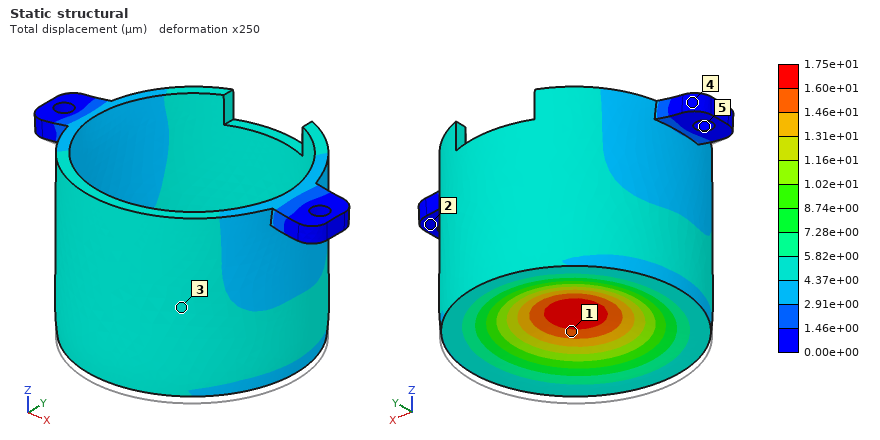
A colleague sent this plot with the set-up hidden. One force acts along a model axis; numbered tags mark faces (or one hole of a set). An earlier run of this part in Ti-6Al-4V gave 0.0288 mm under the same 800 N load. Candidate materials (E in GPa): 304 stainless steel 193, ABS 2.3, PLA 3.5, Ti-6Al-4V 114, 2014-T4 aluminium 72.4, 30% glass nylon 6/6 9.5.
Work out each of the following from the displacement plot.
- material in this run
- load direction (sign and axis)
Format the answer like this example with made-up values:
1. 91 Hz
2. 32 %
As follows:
1. 304 stainless steel
2. +Z
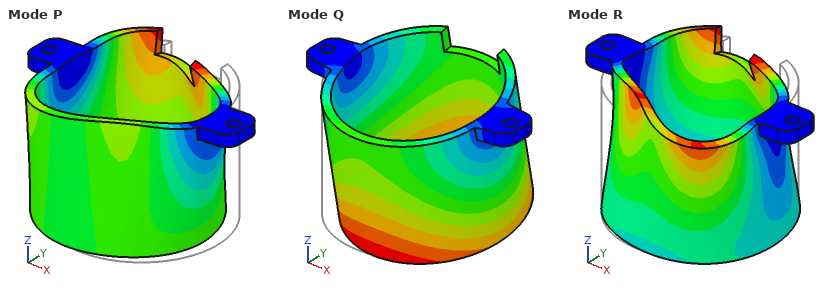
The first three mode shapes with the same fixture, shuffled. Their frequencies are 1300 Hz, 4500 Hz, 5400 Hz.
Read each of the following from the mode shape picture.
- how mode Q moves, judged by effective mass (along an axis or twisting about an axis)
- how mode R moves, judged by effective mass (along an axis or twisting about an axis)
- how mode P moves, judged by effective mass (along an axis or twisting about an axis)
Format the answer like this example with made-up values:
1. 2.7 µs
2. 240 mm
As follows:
1. along Y
2. twisting about Z
3. along X
